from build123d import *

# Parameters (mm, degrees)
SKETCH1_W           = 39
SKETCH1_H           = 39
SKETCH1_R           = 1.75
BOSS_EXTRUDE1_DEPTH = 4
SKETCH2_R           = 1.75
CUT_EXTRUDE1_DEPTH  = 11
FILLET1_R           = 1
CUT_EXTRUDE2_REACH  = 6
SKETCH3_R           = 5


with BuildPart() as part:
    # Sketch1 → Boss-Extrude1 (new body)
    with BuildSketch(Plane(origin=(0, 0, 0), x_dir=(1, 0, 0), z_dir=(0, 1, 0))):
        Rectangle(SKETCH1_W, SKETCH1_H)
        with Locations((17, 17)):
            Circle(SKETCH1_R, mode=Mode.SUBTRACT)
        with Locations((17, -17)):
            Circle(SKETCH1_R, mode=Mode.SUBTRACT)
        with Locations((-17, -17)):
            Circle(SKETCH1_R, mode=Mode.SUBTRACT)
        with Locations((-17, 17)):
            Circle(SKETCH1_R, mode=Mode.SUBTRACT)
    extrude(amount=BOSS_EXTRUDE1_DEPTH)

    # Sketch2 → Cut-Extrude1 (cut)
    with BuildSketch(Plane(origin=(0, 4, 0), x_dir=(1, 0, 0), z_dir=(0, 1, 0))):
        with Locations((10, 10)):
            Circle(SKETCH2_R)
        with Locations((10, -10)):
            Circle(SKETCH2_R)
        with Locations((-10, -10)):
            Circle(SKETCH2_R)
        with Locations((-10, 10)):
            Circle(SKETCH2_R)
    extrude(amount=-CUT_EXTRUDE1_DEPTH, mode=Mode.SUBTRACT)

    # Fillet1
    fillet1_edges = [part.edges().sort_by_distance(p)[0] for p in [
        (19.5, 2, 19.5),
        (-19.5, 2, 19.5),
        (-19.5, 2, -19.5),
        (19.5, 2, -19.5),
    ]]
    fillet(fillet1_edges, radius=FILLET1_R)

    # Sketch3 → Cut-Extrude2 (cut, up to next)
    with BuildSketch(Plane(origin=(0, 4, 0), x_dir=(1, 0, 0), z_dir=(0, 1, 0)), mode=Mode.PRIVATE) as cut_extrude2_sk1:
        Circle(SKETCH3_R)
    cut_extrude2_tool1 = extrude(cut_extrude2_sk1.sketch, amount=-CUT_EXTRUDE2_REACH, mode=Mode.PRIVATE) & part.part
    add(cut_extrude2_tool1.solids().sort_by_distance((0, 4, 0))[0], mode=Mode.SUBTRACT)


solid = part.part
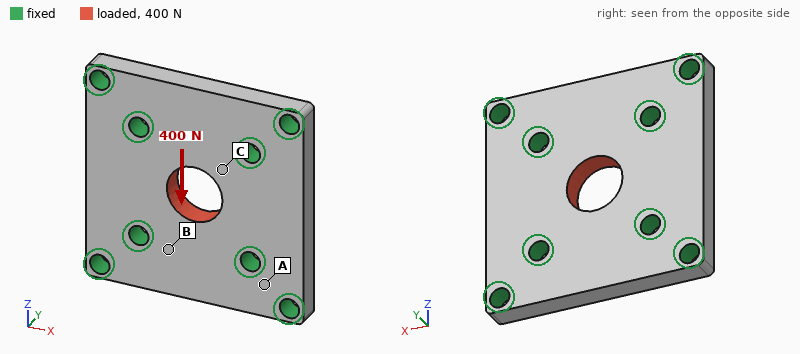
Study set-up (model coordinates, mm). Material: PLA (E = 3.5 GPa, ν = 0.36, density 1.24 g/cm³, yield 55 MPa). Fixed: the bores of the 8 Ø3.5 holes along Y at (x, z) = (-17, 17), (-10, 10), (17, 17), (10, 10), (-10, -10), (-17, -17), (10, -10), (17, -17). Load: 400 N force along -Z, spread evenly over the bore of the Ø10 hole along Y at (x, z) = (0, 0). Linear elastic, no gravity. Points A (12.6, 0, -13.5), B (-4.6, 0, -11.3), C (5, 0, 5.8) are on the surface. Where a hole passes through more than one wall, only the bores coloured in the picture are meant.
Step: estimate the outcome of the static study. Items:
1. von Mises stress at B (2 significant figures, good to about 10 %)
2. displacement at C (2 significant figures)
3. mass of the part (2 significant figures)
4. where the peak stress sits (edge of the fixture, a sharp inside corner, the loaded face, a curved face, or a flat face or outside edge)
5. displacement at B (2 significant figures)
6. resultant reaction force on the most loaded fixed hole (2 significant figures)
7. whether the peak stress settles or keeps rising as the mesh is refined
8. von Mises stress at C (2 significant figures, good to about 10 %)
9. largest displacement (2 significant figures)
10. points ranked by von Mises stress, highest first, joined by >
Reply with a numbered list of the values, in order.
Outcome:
1. 1.9 MPa
2. 6.3 µm
3. 6.8 g
4. edge of the fixture
5. 5.3 µm
6. 97 N
7. keeps rising
8. 2.9 MPa
9. 11 µm
10. C > B > A
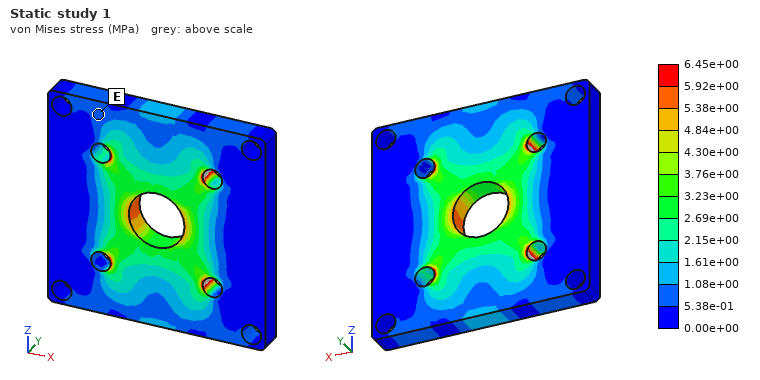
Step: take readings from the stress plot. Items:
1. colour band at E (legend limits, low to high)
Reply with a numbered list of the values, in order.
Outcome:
1. 5.38e-01 to 1.08e+00 MPa
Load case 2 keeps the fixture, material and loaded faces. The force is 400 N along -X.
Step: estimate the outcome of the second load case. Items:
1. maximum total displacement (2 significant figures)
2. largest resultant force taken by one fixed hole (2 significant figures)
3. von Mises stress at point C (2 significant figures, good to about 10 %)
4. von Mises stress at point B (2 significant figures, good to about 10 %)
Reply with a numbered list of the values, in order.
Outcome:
1. 11 µm
2. 97 N
3. 2.9 MPa
4. 0.96 MPa
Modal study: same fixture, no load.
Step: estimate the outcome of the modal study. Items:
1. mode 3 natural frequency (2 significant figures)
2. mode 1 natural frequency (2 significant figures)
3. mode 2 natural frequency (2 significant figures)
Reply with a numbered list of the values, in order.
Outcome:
1. 11 kHz
2. 11 kHz
3. 11 kHz
